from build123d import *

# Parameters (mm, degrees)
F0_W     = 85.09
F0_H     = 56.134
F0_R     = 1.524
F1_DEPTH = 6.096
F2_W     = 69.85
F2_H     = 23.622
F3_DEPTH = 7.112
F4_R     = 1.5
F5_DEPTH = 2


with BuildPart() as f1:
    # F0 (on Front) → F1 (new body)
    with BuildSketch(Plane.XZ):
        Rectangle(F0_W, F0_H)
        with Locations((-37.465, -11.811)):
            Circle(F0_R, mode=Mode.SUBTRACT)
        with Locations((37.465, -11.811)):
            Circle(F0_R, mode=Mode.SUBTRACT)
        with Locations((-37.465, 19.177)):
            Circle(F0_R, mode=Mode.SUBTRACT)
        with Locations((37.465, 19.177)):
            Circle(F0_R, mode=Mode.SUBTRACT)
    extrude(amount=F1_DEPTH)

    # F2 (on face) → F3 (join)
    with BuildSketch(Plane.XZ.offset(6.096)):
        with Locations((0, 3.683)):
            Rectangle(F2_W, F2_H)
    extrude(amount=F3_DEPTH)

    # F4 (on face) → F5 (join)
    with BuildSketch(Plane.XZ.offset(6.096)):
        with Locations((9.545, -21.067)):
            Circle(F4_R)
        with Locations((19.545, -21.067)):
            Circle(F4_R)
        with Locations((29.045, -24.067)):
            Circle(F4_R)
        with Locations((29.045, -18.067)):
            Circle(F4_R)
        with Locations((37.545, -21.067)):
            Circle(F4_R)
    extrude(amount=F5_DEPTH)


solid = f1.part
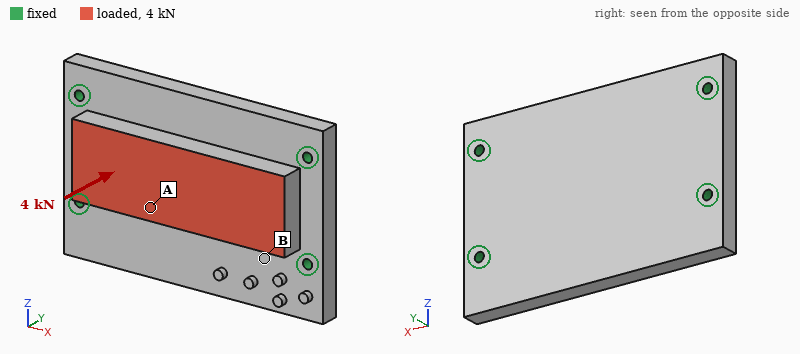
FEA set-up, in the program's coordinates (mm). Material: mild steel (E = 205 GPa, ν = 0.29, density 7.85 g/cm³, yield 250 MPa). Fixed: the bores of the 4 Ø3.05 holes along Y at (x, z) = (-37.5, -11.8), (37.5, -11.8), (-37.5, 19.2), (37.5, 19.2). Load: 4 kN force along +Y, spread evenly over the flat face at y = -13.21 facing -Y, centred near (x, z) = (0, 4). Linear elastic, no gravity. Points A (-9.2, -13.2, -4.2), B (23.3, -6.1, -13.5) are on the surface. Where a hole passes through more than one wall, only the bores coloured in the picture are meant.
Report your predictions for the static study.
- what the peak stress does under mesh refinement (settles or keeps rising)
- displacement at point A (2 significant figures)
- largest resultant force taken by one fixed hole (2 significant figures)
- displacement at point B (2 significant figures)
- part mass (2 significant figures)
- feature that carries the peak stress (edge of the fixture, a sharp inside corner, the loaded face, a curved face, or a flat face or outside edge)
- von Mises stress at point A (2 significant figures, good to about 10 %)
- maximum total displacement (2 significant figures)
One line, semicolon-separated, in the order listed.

keeps rising; 11 µm; 1.3 kN; 6.4 µm; 320 g; edge of the fixture; 28 MPa; 13 µm
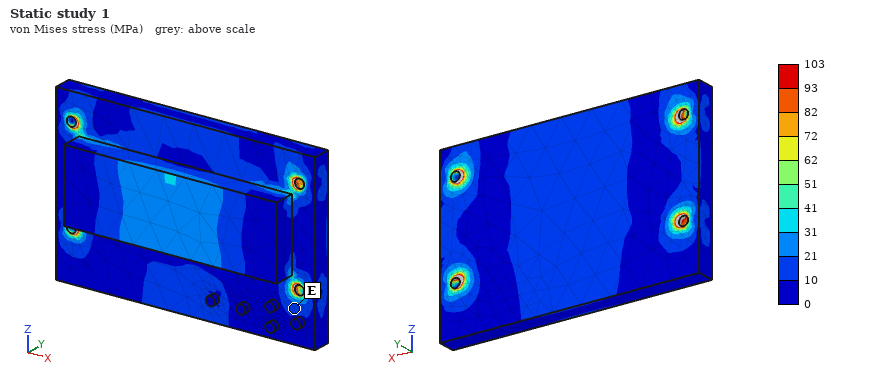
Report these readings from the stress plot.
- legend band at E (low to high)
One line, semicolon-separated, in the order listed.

10 to 21 MPa
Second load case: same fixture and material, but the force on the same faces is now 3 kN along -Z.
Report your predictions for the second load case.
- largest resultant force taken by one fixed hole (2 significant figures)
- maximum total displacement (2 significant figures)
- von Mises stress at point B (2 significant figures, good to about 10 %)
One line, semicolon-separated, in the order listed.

1.0 kN; 5.3 µm; 8.9 MPa
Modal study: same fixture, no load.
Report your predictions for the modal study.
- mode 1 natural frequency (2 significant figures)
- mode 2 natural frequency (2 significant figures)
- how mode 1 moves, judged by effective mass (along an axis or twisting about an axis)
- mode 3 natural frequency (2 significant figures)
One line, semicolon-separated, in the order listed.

5800 Hz; 8000 Hz; along Y; 13 kHz
